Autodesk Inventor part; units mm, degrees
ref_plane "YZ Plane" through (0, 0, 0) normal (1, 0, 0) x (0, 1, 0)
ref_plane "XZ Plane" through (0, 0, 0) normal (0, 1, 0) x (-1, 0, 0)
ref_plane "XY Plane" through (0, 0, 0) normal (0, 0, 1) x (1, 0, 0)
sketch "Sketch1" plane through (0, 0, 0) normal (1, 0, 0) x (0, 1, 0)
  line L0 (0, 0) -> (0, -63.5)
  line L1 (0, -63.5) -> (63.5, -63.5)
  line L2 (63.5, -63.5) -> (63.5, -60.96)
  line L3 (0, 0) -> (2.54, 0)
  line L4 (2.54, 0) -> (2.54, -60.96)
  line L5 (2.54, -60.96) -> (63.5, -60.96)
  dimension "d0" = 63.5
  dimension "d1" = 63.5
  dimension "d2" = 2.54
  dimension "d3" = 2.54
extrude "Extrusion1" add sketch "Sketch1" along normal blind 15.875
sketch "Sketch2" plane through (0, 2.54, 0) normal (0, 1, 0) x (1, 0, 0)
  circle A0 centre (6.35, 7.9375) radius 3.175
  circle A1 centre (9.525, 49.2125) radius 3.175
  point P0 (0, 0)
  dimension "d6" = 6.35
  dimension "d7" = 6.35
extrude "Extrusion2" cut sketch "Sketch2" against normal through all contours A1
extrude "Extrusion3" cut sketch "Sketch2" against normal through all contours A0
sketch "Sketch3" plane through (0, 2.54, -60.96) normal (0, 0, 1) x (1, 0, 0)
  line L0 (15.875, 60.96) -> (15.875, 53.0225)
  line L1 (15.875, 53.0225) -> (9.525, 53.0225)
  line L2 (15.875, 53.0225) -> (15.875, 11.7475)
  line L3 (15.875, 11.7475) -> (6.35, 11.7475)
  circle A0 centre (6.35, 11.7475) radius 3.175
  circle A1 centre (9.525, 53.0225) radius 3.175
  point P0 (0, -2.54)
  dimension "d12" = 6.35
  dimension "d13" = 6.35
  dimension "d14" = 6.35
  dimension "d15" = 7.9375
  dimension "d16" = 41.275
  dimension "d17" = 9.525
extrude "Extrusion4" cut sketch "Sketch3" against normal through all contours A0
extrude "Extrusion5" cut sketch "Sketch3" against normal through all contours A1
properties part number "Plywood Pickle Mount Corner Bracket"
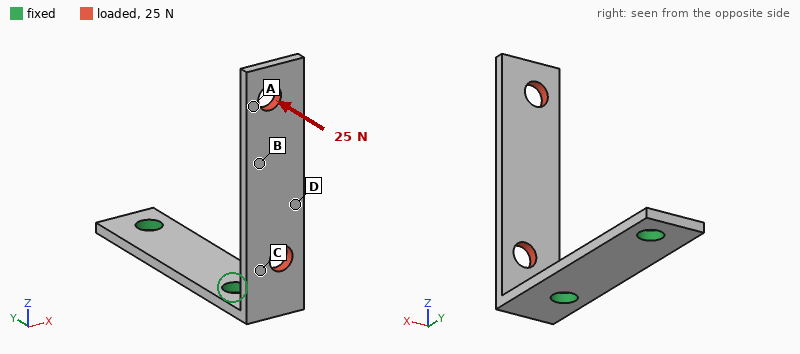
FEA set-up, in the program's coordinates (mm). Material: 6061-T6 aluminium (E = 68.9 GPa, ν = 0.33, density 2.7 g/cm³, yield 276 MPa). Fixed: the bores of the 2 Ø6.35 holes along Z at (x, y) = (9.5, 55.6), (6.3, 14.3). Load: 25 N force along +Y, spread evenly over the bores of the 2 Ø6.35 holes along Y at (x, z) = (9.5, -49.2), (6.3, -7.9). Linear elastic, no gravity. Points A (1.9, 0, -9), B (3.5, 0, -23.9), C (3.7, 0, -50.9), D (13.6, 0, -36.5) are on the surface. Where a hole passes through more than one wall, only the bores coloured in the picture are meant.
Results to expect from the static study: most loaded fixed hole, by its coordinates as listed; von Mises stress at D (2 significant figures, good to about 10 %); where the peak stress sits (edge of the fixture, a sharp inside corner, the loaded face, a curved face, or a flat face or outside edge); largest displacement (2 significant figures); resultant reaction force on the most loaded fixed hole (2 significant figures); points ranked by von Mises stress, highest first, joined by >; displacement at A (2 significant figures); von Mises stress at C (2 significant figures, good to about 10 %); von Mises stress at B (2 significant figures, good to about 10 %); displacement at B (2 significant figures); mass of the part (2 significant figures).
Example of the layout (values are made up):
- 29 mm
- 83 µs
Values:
- (6.3, 14.3)
- 21 MPa
- a flat face or outside edge
- 1.00 mm
- 24 N
- C > D > B > A
- 0.82 mm
- 48 MPa
- 12 MPa
- 0.52 mm
- 13 g
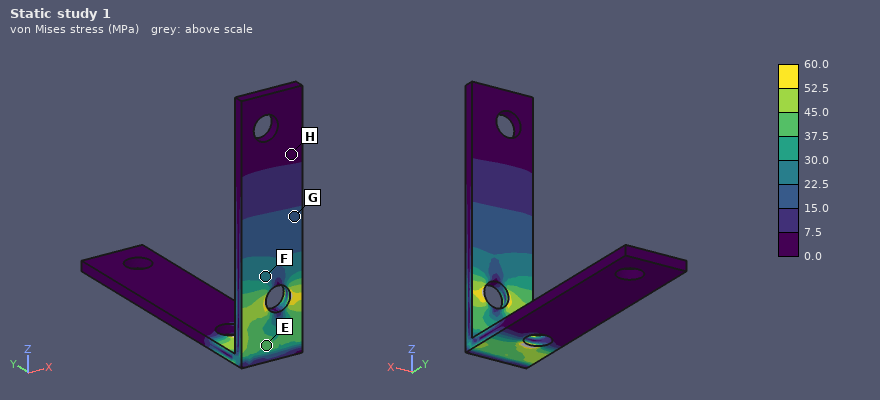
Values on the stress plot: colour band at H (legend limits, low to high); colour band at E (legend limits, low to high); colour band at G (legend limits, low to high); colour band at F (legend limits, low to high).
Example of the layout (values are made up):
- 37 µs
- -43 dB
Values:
- 0.0 to 7.5 MPa
- 37.5 to 45.0 MPa
- 15.0 to 22.5 MPa
- 22.5 to 30.0 MPa
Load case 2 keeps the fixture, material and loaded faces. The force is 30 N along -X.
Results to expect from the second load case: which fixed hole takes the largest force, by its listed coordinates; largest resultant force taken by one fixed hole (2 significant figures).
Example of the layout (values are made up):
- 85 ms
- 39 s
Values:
- (6.3, 14.3)
- 33 N
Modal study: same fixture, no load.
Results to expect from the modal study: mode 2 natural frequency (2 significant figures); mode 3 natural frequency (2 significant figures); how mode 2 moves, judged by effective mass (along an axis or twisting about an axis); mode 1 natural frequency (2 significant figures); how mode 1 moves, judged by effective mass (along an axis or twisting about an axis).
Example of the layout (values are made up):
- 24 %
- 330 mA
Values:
- 880 Hz
- 2700 Hz
- along X
- 420 Hz
- along Y
